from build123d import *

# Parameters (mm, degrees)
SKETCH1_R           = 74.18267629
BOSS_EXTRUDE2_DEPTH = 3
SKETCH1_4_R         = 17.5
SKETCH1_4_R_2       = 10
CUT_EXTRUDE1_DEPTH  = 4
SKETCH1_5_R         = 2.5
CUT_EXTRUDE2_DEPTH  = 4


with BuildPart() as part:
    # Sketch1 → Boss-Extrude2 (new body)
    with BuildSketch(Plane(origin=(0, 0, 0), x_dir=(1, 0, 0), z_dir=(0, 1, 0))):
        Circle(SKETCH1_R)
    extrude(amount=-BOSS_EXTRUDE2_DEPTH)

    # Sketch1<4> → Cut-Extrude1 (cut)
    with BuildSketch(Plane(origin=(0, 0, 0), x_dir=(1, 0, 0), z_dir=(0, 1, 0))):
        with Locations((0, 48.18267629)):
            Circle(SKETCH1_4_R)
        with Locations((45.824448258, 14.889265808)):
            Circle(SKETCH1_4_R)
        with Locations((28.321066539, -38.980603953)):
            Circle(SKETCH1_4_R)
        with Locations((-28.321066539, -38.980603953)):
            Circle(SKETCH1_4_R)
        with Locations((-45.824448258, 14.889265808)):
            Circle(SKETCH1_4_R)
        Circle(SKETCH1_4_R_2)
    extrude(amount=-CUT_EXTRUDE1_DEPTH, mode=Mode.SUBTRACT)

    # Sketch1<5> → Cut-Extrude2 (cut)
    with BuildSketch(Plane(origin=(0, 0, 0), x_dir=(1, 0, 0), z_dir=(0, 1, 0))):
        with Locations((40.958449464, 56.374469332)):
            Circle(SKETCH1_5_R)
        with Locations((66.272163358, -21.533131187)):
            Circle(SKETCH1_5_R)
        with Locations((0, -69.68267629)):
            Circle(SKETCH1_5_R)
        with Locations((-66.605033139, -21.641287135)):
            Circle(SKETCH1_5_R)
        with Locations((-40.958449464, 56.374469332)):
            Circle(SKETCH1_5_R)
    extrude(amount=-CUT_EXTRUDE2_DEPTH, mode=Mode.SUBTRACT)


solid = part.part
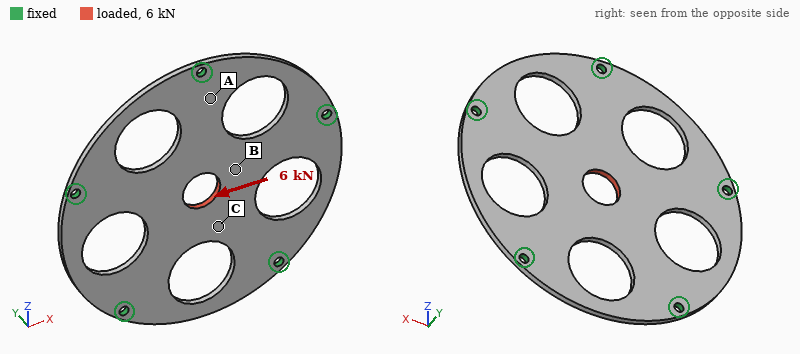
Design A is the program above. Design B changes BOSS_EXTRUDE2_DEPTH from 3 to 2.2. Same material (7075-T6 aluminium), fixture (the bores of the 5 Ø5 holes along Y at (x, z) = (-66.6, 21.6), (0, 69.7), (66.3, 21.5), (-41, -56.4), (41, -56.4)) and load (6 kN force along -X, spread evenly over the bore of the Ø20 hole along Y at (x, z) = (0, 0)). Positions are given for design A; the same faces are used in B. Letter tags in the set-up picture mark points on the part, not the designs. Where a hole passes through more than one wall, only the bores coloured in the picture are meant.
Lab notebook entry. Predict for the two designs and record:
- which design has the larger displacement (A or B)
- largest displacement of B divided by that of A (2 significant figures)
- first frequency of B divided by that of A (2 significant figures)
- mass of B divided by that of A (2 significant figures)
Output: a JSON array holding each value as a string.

["B", "1.4", "0.74", "0.73"]
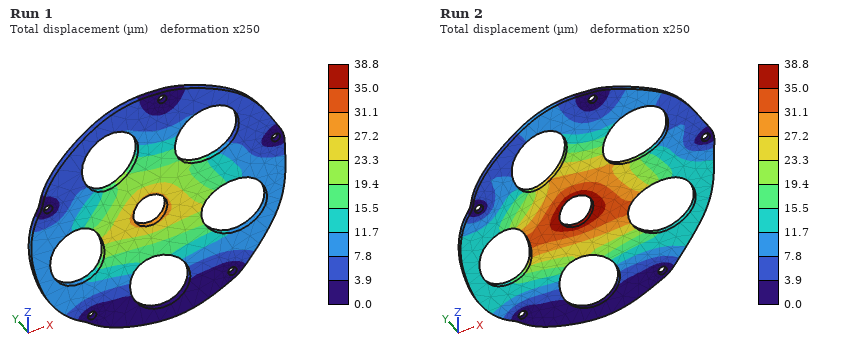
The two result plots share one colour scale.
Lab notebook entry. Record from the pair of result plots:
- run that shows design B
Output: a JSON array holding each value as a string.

["Run 2"]
